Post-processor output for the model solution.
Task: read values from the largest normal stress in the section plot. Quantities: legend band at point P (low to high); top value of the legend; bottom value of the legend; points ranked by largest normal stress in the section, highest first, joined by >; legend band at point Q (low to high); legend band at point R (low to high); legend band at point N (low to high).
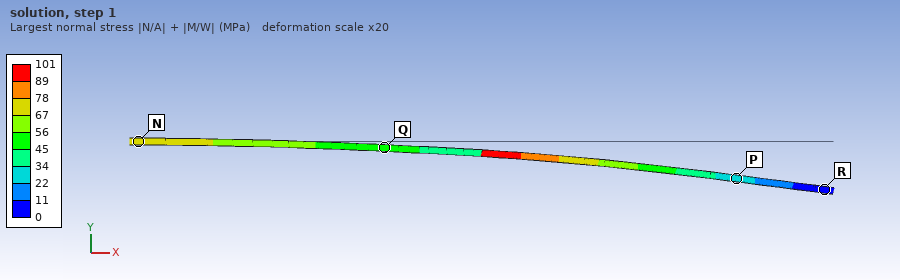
22 to 34 MPa
101 MPa
0 MPa
N > Q > P > R
45 to 56 MPa
0 to 11 MPa
67 to 78 MPa
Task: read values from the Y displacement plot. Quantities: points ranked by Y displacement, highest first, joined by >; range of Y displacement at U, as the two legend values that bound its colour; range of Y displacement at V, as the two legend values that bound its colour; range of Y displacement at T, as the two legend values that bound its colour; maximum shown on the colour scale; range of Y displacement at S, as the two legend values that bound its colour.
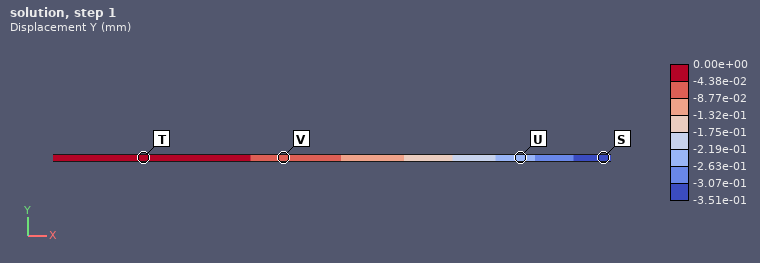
T > V > U > S
-2.63e-01 to -2.19e-01 mm
-8.77e-02 to -4.38e-02 mm
-4.38e-02 to 0.00e+00 mm
0.00e+00 mm
-3.51e-01 to -3.07e-01 mm
